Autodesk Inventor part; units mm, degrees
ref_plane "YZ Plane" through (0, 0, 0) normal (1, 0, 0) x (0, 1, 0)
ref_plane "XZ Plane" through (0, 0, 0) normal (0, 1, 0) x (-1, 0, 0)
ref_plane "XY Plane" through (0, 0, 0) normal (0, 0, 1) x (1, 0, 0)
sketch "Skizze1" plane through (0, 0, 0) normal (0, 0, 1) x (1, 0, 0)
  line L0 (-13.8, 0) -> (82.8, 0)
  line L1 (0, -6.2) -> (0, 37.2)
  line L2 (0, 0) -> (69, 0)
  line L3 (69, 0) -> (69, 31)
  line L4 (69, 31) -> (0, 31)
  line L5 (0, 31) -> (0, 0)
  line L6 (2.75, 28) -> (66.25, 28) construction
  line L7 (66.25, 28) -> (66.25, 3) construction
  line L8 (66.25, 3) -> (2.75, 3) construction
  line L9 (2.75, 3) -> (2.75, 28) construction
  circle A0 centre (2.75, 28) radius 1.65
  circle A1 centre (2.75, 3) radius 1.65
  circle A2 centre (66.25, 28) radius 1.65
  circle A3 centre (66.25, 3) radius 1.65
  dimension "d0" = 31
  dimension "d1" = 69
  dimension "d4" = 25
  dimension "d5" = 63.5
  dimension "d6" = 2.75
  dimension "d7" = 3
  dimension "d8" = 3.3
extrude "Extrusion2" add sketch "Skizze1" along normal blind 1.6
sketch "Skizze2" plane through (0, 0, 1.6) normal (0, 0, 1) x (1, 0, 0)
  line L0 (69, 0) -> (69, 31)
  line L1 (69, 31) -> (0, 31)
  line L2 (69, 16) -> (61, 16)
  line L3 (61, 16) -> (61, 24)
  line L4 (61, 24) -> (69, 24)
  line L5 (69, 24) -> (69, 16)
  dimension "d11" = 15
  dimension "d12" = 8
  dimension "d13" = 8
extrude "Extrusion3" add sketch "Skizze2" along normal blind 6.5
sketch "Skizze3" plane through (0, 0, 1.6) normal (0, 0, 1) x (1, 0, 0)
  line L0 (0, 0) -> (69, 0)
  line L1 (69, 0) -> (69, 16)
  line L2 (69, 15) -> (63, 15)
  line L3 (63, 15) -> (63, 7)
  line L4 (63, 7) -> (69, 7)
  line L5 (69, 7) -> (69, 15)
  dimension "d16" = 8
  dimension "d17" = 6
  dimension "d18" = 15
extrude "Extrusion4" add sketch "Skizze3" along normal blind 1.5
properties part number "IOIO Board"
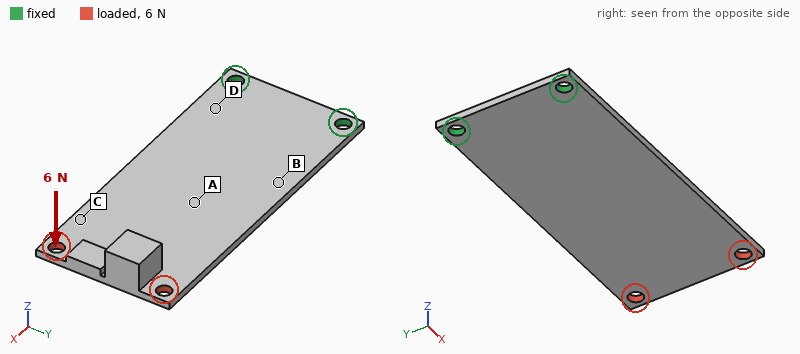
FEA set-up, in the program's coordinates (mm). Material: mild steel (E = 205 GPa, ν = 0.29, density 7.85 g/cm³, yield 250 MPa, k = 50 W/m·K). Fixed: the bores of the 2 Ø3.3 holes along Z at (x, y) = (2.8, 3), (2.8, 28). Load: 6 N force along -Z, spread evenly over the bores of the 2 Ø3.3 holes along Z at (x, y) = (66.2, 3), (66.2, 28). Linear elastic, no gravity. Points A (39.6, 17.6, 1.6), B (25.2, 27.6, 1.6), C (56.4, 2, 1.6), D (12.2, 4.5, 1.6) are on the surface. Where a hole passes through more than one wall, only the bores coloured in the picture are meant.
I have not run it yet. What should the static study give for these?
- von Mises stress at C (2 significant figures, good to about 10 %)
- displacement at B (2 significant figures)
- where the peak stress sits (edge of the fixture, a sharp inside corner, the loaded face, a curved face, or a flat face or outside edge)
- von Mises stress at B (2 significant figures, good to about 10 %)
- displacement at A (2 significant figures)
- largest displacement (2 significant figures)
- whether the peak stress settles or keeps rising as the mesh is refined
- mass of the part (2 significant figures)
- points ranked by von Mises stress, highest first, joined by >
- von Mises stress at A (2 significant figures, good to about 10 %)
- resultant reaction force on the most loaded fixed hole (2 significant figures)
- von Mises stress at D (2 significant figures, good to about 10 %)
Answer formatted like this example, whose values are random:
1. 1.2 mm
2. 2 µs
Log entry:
1. 4.9 MPa
2. 0.041 mm
3. edge of the fixture
4. 19 MPa
5. 0.10 mm
6. 0.26 mm
7. keeps rising
8. 30 g
9. D > B > A > C
10. 12 MPa
11. 3.0 N
12. 24 MPa
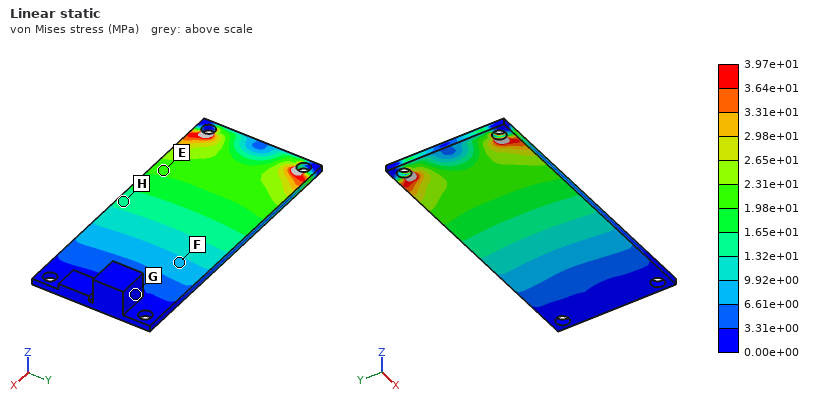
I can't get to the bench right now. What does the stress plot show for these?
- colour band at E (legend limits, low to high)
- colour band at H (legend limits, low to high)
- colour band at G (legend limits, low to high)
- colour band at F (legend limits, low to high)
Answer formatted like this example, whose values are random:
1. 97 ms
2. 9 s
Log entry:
1. 1.98e+01 to 2.31e+01 MPa
2. 1.32e+01 to 1.65e+01 MPa
3. 0.00e+00 to 3.31e+00 MPa
4. 6.61e+00 to 9.92e+00 MPa
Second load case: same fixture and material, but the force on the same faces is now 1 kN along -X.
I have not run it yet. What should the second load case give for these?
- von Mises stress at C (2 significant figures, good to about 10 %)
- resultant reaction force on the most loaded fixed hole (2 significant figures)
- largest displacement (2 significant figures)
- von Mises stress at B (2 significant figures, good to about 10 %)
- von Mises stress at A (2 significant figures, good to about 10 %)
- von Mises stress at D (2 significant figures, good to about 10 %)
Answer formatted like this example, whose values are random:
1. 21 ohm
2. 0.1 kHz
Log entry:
1. 33 MPa
2. 520 N
3. 10 µm
4. 21 MPa
5. 19 MPa
6. 27 MPa
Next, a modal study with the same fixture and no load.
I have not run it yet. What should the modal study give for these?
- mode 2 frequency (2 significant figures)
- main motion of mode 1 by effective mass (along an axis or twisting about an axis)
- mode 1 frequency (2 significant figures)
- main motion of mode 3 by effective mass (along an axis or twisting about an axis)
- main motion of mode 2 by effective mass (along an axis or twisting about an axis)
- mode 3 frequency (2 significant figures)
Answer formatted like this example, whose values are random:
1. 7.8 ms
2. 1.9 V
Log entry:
1. 1300 Hz
2. along Z
3. 240 Hz
4. along Z
5. twisting about X
6. 1700 Hz
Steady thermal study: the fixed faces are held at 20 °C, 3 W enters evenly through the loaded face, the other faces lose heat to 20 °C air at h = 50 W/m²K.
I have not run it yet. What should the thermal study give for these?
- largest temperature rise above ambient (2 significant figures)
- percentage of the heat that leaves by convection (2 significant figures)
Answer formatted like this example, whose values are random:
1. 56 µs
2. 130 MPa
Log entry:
1. 37 K
2. 85 %
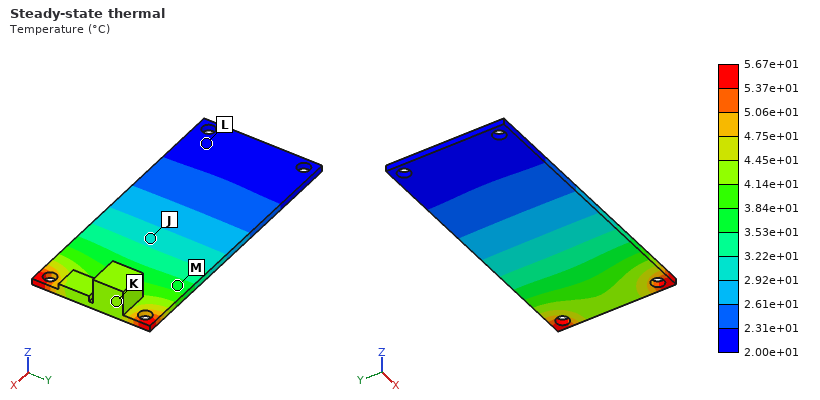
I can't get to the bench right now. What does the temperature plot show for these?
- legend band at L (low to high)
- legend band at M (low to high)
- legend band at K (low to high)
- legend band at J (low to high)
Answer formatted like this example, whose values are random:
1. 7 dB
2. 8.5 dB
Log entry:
1. 2.00e+01 to 2.31e+01 °C
2. 3.53e+01 to 3.84e+01 °C
3. 4.14e+01 to 4.45e+01 °C
4. 2.92e+01 to 3.22e+01 °C
